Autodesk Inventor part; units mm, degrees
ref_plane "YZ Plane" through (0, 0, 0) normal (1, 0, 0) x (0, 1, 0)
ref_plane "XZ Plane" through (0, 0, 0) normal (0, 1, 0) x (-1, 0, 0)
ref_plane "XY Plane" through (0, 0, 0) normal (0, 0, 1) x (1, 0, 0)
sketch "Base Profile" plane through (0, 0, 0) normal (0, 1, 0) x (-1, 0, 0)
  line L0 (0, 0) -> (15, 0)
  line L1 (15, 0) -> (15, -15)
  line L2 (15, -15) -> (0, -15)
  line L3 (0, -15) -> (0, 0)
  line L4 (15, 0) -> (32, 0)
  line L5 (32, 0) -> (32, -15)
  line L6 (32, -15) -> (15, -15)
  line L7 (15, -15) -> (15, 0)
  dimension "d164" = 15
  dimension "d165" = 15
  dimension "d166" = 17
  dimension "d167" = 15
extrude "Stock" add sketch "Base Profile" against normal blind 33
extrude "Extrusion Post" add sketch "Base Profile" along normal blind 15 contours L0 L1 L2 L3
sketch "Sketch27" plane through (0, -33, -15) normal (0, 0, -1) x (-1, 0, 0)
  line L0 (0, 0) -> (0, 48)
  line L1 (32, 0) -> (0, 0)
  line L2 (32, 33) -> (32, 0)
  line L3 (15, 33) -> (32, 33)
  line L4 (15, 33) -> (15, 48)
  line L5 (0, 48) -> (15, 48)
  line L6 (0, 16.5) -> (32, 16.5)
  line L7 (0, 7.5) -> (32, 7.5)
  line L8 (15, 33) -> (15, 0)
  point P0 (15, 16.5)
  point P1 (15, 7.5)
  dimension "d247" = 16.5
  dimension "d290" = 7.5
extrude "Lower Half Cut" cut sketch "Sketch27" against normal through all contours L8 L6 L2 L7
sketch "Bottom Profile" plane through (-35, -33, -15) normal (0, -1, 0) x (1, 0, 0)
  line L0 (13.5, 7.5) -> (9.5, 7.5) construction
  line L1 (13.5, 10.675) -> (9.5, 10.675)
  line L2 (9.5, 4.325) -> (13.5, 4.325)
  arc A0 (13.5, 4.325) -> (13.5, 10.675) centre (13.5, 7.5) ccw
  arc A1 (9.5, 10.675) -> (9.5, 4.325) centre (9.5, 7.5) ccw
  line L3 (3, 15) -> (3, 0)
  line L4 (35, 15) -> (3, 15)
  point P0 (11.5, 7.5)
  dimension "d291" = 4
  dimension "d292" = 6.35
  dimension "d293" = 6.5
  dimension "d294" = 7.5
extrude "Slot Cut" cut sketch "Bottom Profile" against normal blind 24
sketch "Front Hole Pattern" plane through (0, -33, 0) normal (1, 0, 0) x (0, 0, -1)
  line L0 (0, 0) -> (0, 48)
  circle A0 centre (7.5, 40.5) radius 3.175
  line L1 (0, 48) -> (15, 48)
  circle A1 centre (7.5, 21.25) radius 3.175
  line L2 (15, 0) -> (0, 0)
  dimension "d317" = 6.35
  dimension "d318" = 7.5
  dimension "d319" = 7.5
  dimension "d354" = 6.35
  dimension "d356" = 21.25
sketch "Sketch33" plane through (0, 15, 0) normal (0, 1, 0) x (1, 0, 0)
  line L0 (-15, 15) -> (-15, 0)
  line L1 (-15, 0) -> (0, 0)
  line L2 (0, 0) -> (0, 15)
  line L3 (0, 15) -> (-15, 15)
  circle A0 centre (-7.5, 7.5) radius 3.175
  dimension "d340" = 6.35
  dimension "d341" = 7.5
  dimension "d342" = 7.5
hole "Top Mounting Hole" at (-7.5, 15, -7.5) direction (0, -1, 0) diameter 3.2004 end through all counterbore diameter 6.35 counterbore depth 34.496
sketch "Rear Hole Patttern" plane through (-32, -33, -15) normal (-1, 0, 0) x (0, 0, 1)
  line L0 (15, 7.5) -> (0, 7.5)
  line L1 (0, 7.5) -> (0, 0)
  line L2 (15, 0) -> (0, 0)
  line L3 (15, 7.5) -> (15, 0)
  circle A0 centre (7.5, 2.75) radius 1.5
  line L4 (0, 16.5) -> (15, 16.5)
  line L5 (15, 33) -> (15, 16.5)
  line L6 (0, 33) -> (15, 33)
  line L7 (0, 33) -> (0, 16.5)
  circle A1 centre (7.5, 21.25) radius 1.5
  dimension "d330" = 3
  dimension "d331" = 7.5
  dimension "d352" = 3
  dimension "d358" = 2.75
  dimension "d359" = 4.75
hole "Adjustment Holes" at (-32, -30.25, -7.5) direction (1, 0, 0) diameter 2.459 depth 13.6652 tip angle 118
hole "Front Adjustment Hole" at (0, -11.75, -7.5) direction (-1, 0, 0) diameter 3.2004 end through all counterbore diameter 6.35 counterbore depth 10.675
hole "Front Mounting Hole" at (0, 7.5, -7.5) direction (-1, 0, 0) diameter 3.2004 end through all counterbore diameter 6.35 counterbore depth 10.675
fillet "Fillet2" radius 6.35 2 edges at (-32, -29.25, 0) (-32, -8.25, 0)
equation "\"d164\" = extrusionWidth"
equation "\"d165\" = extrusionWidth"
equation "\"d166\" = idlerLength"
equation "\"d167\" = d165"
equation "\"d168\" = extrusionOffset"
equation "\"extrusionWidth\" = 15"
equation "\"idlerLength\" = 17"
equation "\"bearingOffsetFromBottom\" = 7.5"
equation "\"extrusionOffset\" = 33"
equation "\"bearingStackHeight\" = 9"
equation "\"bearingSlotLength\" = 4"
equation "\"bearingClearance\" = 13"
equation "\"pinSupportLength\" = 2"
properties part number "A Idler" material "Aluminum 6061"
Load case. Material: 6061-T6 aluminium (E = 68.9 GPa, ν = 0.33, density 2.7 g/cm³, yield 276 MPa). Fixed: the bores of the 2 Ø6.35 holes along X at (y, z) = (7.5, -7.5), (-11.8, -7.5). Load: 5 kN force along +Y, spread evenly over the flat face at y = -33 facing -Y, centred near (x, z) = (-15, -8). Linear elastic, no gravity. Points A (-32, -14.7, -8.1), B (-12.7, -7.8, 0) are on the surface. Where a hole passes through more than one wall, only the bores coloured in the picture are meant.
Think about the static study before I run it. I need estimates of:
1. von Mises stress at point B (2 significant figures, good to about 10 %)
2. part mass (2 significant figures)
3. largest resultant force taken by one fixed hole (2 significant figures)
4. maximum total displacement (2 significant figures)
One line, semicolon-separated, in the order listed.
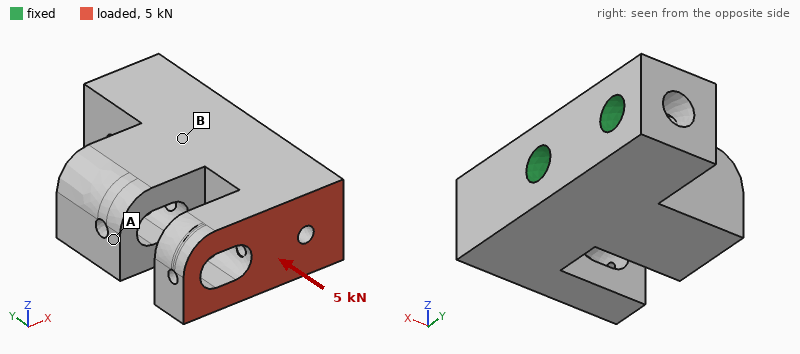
45 MPa; 38 g; 3.3 kN; 0.21 mm
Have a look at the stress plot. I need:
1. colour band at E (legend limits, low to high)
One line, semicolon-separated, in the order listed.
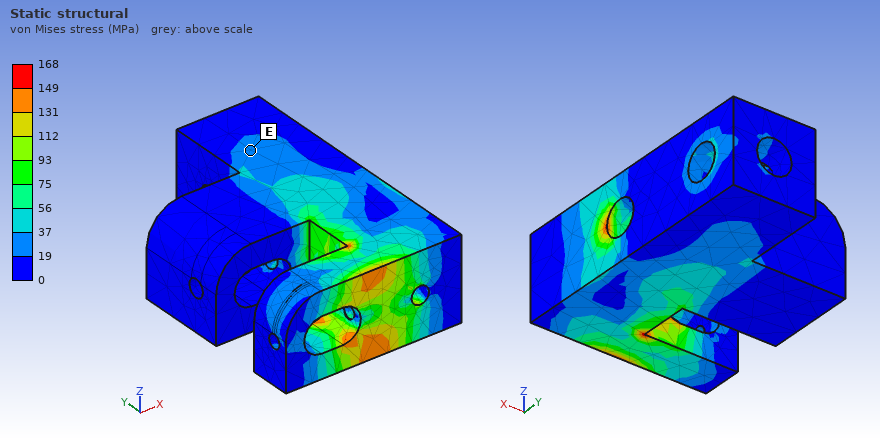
19 to 37 MPa
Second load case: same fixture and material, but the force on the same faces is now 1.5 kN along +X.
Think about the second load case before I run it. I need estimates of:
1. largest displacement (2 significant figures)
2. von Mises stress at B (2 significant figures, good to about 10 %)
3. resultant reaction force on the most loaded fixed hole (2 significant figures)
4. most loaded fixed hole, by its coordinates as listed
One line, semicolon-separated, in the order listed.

72 µm; 22 MPa; 2.7 kN; (-11.8, -7.5)
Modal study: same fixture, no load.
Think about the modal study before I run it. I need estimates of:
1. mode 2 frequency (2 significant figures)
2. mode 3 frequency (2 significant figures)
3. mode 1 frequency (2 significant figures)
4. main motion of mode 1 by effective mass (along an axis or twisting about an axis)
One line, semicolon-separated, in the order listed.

9300 Hz; 12 kHz; 7900 Hz; along Z
